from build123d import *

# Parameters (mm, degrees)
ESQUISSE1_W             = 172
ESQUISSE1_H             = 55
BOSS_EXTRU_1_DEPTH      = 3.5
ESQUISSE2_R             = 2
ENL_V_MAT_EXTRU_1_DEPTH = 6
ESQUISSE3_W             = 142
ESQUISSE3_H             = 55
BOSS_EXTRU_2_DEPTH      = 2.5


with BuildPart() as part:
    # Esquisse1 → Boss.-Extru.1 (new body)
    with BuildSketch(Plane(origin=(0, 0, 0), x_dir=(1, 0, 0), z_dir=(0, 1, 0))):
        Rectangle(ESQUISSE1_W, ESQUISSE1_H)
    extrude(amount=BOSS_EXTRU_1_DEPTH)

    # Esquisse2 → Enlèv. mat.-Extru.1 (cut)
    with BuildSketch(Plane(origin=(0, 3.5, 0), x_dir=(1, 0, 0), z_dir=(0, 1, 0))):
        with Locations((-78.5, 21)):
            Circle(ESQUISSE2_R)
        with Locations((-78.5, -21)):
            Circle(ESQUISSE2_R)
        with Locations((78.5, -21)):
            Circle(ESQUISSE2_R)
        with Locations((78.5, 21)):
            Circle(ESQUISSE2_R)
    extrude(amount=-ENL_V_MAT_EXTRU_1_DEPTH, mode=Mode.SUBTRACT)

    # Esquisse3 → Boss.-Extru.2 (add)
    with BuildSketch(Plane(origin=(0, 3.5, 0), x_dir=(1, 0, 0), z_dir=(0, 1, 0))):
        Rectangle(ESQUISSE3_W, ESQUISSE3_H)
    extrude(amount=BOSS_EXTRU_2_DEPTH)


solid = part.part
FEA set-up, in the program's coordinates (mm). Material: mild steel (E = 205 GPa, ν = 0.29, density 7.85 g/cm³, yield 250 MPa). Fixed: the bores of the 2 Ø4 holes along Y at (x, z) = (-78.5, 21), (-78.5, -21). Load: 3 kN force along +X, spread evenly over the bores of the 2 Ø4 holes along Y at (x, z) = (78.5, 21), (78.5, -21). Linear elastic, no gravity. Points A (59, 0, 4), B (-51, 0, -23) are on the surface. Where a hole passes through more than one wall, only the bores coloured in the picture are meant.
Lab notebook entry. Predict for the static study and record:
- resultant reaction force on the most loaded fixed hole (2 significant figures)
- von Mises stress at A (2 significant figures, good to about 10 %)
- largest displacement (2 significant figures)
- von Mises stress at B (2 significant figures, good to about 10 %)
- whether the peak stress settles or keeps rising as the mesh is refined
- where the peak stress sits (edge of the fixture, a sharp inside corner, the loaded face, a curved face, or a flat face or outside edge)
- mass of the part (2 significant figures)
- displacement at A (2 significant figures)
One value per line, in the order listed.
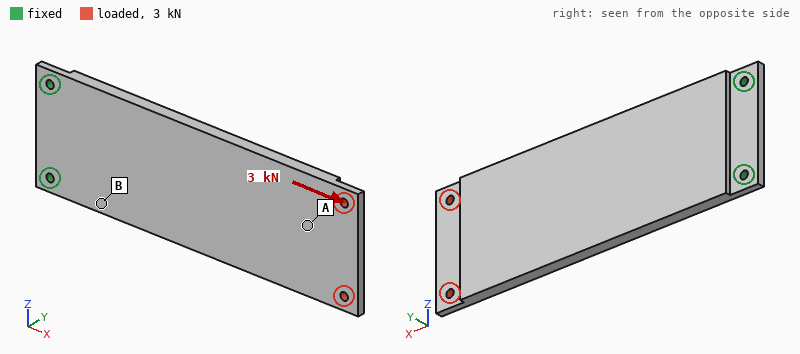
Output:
1.5 kN
15 MPa
0.22 mm
22 MPa
keeps rising
edge of the fixture
410 g
0.15 mm
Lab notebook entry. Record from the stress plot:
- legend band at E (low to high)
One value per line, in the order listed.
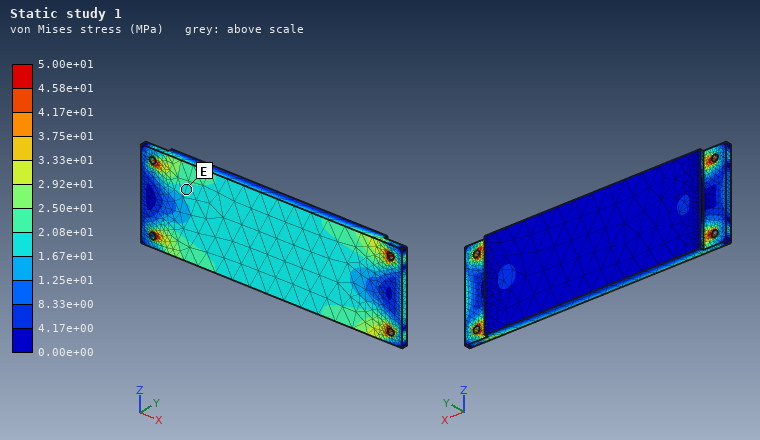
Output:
1.67e+01 to 2.08e+01 MPa
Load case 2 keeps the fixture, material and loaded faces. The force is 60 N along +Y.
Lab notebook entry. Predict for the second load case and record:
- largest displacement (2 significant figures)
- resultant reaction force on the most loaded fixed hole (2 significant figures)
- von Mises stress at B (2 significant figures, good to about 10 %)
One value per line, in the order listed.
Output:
0.75 mm
59 N
23 MPa
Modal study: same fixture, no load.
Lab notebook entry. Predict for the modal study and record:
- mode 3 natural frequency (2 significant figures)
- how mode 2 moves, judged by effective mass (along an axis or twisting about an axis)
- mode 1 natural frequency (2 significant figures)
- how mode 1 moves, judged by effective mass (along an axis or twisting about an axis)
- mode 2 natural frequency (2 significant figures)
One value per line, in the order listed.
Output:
1100 Hz
along Y
140 Hz
along Y
1000 Hz
